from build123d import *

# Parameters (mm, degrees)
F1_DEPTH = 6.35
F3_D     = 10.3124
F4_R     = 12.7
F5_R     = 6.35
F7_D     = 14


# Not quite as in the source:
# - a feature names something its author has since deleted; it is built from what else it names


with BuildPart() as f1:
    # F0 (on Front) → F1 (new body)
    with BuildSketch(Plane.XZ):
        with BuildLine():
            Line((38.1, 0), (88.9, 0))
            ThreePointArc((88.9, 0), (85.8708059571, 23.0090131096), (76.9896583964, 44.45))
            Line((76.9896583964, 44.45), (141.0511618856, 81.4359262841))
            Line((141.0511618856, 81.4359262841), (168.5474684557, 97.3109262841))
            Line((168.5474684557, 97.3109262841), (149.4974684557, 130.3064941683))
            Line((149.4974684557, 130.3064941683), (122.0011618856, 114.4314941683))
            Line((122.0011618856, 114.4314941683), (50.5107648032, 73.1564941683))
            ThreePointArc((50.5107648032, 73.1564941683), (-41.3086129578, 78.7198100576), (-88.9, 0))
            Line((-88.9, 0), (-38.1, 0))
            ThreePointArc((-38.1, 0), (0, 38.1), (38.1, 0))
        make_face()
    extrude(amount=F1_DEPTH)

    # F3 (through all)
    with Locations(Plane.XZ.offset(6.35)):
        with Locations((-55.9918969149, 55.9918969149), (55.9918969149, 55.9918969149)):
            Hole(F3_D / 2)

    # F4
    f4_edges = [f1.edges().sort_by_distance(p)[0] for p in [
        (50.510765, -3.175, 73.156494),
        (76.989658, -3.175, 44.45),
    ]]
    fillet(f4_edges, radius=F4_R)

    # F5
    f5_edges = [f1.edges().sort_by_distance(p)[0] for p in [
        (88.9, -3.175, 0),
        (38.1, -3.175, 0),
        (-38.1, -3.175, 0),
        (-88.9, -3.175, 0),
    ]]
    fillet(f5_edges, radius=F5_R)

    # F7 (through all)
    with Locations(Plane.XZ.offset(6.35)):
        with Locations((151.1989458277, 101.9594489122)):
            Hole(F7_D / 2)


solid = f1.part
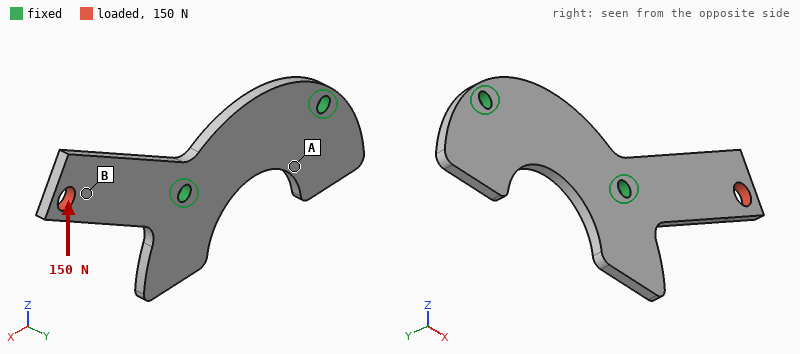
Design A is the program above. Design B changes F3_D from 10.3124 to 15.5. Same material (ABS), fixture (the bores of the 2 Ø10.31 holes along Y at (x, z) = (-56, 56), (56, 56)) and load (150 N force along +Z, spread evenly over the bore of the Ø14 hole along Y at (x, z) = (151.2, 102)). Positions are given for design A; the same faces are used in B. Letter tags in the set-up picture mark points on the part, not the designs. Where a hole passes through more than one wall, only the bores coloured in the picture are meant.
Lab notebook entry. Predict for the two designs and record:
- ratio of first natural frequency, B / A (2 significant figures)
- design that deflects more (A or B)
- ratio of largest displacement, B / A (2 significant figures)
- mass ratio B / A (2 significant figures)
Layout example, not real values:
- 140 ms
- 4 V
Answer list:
- 1.1
- A
- 0.89
- 0.98
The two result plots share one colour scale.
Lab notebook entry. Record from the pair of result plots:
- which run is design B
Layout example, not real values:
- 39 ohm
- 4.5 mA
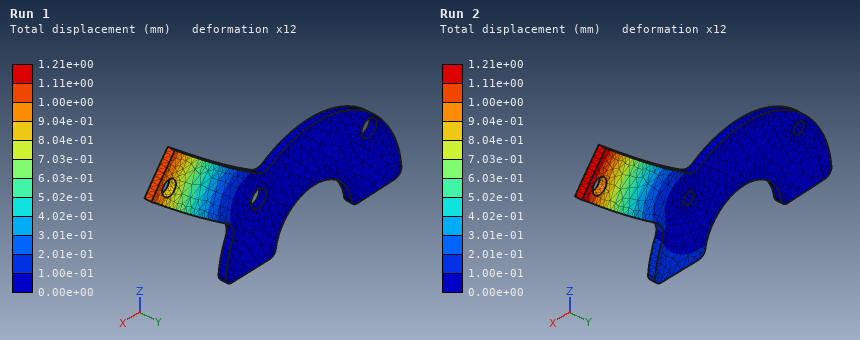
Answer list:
- Run 1
